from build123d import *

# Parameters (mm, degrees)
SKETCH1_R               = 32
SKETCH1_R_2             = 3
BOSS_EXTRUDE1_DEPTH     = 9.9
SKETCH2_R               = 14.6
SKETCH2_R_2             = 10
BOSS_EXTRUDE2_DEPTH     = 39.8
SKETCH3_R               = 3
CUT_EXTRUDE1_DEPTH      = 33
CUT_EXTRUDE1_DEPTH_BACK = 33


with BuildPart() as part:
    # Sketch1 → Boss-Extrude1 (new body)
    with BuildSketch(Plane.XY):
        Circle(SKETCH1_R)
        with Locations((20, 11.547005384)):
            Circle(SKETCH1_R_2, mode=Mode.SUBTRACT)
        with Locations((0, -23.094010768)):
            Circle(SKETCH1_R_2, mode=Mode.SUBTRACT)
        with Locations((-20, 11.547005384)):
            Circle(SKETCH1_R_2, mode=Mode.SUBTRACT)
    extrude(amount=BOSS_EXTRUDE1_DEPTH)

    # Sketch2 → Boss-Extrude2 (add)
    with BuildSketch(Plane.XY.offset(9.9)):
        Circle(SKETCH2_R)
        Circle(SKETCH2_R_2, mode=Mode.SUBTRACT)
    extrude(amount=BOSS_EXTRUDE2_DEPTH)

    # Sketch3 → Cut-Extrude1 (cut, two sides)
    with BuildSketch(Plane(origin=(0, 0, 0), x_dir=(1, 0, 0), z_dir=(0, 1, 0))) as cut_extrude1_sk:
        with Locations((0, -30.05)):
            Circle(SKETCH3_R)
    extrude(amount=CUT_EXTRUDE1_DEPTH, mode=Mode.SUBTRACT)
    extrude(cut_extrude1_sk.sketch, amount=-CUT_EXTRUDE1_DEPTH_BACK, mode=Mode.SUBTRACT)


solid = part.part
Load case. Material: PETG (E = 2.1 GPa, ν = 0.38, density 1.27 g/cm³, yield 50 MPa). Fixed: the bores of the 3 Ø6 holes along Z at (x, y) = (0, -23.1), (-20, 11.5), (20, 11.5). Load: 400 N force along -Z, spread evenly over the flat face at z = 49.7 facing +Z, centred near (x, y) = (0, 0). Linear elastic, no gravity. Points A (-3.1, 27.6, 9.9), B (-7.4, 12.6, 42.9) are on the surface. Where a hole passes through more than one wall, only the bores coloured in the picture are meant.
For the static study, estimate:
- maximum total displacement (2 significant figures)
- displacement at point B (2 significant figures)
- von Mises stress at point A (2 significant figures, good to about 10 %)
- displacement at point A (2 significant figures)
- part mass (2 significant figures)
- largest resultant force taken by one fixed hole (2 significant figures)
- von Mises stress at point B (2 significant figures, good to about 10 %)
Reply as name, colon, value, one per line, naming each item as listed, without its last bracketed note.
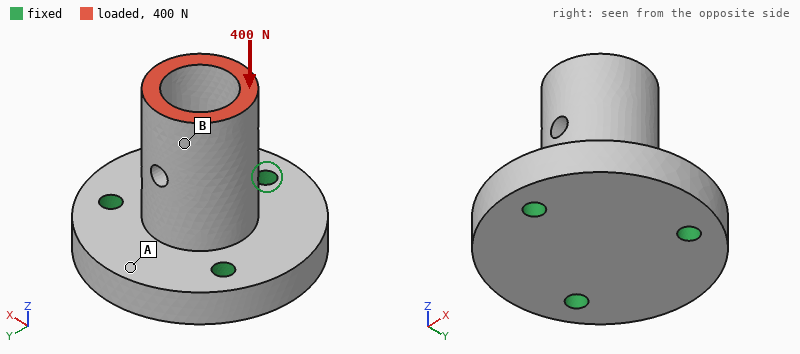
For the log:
maximum total displacement: 38 µm
displacement at point B: 34 µm
von Mises stress at point A: 0.44 MPa
displacement at point A: 8.6 µm
part mass: 57 g
largest resultant force taken by one fixed hole: 140 N
von Mises stress at point B: 1.2 MPa
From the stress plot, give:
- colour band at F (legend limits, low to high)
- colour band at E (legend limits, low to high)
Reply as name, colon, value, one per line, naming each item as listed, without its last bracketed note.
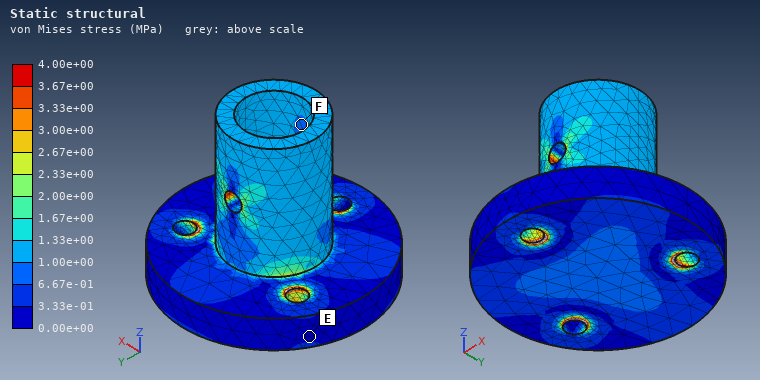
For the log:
colour band at F: 6.67e-01 to 1.00e+00 MPa
colour band at E: 0.00e+00 to 3.33e-01 MPa
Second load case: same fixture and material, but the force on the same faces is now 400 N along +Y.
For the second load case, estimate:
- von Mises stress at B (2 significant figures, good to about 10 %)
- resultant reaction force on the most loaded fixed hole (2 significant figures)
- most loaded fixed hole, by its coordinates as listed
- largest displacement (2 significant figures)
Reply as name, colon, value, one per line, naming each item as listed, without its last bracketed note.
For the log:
von Mises stress at B: 3.0 MPa
resultant reaction force on the most loaded fixed hole: 520 N
most loaded fixed hole, by its coordinates as listed: (0, -23.1)
largest displacement: 0.46 mm
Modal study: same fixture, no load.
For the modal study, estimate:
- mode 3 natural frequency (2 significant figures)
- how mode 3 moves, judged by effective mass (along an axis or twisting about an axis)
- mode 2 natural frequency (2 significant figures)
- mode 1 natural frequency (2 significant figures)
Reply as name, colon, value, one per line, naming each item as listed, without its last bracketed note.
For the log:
mode 3 natural frequency: 3900 Hz
how mode 3 moves, judged by effective mass: along Z
mode 2 natural frequency: 2000 Hz
mode 1 natural frequency: 1900 Hz
